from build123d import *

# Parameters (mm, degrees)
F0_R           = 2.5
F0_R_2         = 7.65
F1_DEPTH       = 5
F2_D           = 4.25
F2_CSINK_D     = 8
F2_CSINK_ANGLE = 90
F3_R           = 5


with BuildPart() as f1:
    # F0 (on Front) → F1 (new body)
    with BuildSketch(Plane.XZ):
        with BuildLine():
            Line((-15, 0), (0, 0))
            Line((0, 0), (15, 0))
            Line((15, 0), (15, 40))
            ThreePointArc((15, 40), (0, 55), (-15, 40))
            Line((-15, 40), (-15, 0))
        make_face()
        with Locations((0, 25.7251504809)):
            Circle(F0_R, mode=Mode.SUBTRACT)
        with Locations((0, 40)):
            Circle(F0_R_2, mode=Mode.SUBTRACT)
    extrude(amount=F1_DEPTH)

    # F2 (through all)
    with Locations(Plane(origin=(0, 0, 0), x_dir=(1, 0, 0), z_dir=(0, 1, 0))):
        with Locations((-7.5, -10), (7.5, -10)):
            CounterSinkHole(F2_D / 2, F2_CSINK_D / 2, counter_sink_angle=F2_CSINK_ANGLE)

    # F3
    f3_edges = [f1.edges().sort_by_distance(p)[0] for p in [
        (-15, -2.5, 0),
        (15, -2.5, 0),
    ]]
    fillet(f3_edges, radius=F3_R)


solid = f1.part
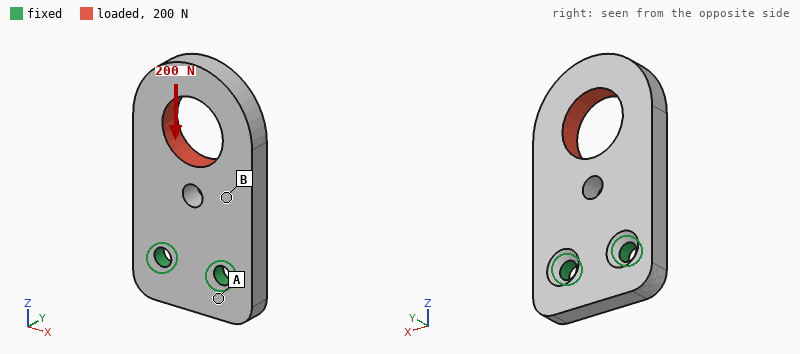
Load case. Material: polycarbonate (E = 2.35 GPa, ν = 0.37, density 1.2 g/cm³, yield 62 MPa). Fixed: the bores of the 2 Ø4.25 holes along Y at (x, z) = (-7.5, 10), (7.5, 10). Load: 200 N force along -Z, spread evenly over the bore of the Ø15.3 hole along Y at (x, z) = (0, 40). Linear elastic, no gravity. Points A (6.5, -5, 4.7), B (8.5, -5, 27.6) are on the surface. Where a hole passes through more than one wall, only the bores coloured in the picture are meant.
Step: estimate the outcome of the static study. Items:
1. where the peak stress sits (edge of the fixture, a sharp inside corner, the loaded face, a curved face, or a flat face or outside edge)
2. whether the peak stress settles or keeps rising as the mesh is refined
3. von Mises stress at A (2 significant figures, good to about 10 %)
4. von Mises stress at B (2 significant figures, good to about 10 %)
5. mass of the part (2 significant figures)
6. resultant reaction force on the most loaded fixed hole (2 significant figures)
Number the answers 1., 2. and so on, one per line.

1. edge of the fixture
2. keeps rising
3. 0.59 MPa
4. 1.6 MPa
5. 7.8 g
6. 100 N
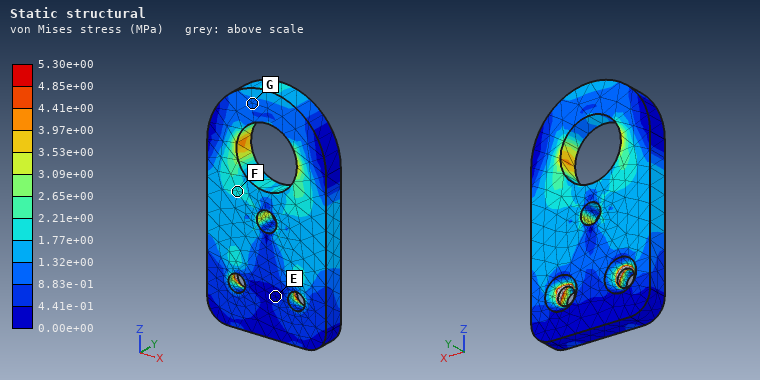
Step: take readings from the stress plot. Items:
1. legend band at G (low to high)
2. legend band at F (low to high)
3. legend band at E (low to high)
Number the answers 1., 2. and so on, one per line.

1. 8.83e-01 to 1.32e+00 MPa
2. 1.77e+00 to 2.21e+00 MPa
3. 0.00e+00 to 4.41e-01 MPa
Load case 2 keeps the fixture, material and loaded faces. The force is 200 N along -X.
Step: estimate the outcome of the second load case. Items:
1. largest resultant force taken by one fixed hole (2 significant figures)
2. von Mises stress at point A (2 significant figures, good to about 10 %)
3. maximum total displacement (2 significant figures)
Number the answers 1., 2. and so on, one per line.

1. 350 N
2. 2.7 MPa
3. 0.32 mm
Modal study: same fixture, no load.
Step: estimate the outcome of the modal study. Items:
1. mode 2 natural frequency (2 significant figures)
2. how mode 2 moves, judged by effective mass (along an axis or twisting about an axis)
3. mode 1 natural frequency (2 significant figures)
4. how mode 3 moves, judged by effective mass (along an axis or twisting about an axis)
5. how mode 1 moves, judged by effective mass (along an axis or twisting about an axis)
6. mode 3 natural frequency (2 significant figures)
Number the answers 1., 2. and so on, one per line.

1. 1800 Hz
2. twisting about Z
3. 640 Hz
4. along X
5. along Y
6. 2500 Hz
